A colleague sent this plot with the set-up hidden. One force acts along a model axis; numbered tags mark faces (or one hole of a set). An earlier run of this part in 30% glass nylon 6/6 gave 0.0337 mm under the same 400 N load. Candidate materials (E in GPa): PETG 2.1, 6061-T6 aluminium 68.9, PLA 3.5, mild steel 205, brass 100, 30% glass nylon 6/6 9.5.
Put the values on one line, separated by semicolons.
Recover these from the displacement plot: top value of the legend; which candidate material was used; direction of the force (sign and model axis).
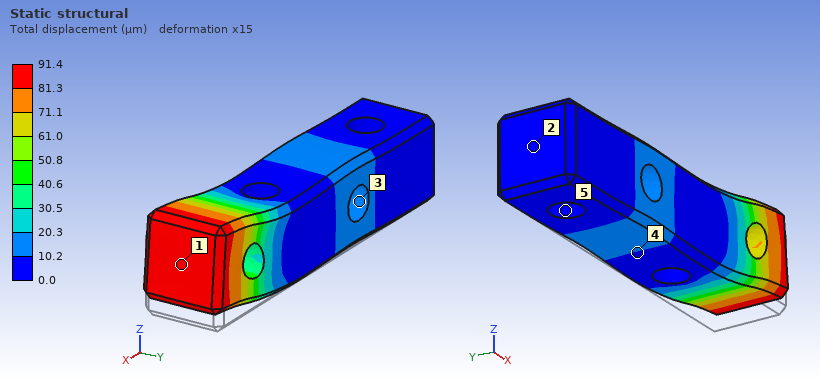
91.4 µm; PLA; +Z
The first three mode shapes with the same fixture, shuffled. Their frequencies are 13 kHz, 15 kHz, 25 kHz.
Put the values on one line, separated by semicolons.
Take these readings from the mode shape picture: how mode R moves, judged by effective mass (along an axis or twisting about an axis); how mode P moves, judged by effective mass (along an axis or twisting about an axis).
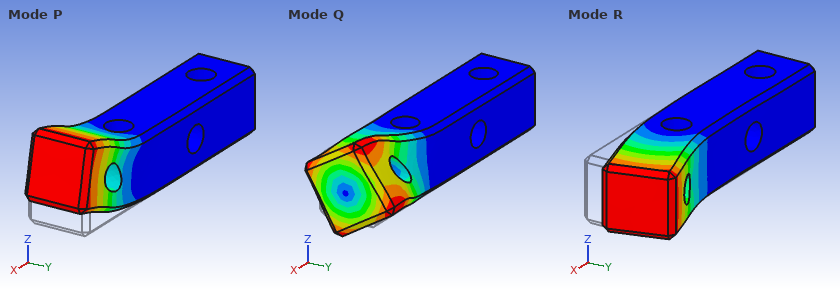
along Y; along Z
